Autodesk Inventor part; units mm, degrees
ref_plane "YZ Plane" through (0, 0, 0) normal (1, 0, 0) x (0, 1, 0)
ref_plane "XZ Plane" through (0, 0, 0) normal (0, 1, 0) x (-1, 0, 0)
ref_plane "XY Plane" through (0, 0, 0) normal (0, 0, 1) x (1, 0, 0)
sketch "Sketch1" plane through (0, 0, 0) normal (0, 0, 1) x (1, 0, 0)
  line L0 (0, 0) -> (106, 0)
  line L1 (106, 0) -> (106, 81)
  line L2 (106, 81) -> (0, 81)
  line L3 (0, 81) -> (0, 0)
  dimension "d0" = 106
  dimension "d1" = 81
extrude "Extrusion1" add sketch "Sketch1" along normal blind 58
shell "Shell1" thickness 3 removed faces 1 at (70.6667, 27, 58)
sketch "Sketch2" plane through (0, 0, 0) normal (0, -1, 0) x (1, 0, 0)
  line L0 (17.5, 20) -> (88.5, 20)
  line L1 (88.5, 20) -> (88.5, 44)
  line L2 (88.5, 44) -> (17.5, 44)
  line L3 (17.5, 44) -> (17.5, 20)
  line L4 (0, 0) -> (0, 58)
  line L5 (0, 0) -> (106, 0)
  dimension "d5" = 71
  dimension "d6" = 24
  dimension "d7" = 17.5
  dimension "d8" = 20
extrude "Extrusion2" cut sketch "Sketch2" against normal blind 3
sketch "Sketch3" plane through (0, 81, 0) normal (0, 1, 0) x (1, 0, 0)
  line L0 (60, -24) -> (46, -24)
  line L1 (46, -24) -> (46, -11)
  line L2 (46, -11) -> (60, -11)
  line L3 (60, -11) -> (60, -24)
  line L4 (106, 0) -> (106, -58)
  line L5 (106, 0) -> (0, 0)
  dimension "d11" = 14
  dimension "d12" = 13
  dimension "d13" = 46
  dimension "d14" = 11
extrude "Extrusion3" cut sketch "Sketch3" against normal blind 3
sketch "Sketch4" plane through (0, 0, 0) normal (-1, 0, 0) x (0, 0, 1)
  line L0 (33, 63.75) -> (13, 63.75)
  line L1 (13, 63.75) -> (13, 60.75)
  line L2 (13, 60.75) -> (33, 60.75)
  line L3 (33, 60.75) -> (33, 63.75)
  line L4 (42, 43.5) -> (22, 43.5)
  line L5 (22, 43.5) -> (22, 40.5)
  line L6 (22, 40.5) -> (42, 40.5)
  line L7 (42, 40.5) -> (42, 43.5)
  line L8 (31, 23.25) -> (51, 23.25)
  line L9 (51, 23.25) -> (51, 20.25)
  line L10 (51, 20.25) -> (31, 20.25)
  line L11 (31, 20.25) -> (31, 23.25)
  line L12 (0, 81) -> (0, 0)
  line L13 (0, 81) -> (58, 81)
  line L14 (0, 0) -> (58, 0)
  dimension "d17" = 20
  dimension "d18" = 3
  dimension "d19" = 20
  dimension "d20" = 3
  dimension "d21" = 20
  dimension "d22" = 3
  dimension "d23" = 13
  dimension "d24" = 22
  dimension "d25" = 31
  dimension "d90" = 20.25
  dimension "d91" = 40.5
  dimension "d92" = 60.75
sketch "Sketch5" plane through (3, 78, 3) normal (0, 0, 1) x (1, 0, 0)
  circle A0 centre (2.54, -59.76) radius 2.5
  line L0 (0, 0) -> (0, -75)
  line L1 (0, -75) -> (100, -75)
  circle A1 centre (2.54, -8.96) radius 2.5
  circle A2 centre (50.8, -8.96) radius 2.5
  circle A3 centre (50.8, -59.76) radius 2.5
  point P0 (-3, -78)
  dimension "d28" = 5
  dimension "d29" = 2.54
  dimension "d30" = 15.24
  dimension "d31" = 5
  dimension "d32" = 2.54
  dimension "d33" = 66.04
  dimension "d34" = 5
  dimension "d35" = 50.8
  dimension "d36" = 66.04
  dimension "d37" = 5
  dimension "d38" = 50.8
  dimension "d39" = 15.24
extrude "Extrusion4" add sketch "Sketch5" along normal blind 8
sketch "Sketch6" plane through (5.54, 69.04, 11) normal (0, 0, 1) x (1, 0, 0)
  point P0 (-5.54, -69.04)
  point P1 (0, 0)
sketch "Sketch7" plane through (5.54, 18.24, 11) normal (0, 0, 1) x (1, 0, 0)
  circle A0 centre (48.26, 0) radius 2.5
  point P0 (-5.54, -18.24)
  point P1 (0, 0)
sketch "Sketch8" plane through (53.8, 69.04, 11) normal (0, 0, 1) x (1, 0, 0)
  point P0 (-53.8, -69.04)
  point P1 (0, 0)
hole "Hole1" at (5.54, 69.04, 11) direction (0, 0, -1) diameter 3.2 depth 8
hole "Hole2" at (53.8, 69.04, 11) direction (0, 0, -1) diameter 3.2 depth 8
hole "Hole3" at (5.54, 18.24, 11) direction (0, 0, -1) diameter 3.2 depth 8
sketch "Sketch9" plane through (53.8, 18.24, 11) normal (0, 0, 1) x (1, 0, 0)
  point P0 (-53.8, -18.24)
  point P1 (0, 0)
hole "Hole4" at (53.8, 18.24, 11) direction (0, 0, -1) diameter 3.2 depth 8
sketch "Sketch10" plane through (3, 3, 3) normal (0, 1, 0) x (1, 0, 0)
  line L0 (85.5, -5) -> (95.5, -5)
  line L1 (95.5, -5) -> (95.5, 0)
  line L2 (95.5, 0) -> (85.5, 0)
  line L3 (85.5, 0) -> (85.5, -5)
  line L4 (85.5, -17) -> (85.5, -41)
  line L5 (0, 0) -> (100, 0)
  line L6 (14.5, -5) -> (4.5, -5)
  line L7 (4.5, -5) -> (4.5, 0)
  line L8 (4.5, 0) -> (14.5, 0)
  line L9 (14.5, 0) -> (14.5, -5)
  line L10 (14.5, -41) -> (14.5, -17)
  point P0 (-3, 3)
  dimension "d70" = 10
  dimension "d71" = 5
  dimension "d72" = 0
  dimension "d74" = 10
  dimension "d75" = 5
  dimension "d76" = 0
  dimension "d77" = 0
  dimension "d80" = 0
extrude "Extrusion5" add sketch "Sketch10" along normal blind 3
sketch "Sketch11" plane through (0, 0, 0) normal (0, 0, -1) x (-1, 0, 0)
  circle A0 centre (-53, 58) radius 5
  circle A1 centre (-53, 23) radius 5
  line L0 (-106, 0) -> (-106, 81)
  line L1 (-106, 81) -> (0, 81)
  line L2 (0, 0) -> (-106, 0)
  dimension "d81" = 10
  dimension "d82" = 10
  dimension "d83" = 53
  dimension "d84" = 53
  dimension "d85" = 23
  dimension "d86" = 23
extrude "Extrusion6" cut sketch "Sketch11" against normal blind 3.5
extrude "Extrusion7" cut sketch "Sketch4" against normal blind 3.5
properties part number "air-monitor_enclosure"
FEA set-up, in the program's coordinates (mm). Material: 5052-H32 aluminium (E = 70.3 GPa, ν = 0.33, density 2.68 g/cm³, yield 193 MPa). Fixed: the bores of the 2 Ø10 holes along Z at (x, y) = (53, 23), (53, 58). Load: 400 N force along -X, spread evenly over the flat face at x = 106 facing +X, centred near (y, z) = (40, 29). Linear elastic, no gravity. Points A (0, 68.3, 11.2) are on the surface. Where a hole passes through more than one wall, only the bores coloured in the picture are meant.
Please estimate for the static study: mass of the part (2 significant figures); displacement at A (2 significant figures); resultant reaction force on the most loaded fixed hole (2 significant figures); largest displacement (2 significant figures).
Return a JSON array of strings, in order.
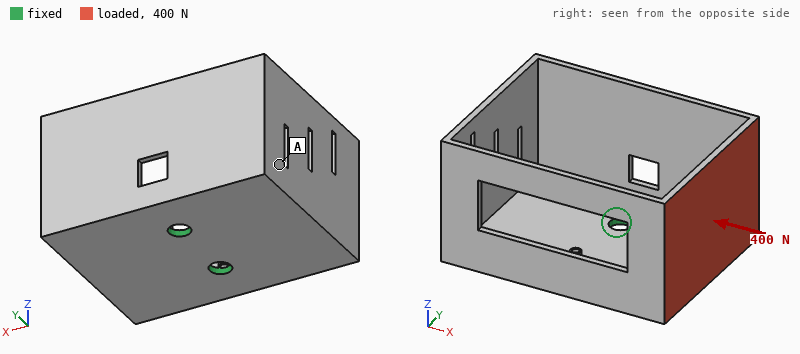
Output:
["210 g", "0.20 mm", "210 N", "0.38 mm"]
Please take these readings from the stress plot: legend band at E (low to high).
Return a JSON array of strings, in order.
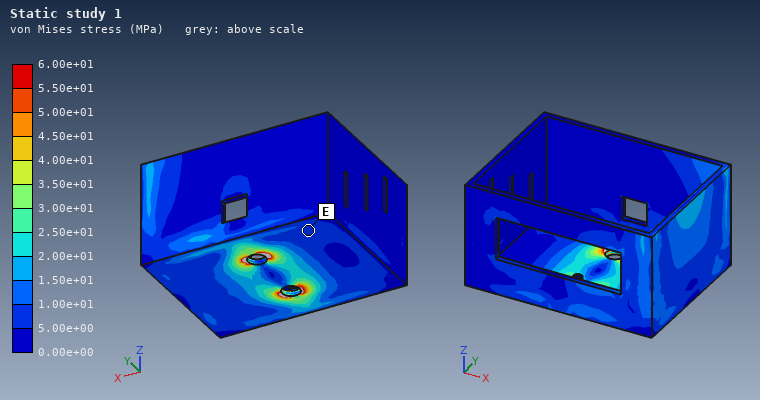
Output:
["5.00e+00 to 1.00e+01 MPa"]
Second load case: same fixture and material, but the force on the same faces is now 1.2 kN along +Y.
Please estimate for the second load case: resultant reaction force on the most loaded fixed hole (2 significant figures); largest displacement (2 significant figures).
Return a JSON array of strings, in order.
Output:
["1.7 kN", "0.73 mm"]
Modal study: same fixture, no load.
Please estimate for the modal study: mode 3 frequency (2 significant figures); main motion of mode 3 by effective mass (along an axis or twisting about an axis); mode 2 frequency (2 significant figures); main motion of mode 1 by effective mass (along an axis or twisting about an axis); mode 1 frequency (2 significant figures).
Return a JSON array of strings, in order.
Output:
["840 Hz", "along Y", "670 Hz", "along X", "400 Hz"]
